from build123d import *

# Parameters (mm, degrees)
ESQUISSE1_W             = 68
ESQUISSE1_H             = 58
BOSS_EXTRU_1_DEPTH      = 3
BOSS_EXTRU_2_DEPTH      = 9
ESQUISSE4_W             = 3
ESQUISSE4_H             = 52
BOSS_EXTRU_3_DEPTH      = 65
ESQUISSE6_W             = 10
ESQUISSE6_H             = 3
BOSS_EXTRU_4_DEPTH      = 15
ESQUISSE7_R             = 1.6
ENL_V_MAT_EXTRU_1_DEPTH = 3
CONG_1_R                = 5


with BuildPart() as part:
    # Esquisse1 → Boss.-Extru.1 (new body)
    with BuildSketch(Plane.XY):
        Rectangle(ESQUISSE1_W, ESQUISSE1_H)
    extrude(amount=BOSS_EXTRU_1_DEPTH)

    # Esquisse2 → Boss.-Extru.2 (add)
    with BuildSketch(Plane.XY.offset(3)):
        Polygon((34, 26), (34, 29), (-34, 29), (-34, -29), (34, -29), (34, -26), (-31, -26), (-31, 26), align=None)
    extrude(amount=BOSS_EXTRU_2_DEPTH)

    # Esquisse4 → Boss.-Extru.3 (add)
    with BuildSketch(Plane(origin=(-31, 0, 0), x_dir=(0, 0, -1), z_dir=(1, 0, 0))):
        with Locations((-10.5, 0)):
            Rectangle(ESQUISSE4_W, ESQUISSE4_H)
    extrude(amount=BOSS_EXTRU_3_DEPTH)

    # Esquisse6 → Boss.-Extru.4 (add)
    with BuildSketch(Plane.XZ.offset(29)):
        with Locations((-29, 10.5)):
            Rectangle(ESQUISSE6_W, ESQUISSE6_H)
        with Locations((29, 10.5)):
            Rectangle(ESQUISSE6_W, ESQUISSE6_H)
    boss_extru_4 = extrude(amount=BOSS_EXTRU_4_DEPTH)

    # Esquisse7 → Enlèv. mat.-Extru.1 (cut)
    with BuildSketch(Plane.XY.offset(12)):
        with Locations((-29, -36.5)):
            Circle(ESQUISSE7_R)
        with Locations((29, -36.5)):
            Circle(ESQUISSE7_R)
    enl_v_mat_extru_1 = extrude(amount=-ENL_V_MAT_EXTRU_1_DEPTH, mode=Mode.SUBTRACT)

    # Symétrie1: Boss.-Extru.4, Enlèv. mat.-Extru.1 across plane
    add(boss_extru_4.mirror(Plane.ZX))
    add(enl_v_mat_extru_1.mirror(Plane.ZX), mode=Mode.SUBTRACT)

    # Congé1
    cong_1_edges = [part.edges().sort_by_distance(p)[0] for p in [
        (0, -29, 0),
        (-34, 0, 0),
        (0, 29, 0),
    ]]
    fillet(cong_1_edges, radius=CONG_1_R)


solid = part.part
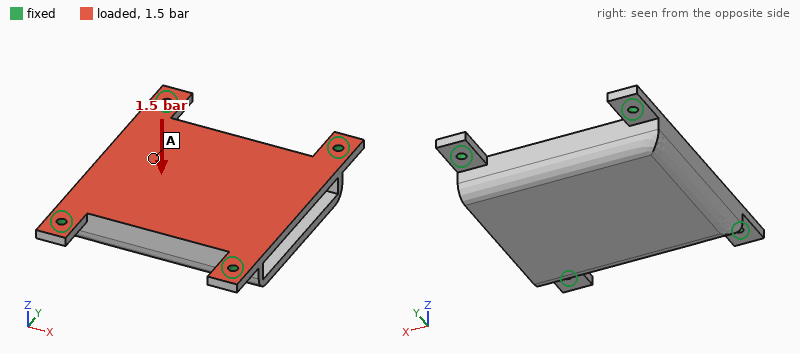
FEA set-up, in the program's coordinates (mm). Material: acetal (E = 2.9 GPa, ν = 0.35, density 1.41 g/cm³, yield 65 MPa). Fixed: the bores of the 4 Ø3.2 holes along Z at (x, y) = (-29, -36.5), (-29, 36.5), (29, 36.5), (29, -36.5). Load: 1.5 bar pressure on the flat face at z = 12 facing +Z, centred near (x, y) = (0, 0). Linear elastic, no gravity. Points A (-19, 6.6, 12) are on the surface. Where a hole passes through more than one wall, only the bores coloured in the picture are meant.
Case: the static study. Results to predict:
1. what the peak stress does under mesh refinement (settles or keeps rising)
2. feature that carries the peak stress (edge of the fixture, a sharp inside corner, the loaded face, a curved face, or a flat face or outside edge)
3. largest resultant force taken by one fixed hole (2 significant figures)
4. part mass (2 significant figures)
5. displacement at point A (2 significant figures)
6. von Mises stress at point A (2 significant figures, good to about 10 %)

keeps rising
edge of the fixture
200 N
39 g
0.51 mm
6.4 MPa
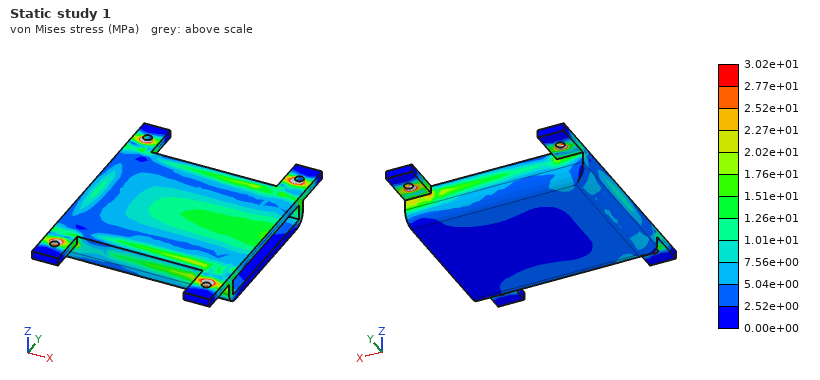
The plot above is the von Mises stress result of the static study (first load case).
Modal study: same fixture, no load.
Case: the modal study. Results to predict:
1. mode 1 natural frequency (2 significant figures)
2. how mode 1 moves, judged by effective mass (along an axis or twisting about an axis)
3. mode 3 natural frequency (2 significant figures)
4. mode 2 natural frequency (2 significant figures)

1000 Hz
along Z
1400 Hz
1300 Hz
